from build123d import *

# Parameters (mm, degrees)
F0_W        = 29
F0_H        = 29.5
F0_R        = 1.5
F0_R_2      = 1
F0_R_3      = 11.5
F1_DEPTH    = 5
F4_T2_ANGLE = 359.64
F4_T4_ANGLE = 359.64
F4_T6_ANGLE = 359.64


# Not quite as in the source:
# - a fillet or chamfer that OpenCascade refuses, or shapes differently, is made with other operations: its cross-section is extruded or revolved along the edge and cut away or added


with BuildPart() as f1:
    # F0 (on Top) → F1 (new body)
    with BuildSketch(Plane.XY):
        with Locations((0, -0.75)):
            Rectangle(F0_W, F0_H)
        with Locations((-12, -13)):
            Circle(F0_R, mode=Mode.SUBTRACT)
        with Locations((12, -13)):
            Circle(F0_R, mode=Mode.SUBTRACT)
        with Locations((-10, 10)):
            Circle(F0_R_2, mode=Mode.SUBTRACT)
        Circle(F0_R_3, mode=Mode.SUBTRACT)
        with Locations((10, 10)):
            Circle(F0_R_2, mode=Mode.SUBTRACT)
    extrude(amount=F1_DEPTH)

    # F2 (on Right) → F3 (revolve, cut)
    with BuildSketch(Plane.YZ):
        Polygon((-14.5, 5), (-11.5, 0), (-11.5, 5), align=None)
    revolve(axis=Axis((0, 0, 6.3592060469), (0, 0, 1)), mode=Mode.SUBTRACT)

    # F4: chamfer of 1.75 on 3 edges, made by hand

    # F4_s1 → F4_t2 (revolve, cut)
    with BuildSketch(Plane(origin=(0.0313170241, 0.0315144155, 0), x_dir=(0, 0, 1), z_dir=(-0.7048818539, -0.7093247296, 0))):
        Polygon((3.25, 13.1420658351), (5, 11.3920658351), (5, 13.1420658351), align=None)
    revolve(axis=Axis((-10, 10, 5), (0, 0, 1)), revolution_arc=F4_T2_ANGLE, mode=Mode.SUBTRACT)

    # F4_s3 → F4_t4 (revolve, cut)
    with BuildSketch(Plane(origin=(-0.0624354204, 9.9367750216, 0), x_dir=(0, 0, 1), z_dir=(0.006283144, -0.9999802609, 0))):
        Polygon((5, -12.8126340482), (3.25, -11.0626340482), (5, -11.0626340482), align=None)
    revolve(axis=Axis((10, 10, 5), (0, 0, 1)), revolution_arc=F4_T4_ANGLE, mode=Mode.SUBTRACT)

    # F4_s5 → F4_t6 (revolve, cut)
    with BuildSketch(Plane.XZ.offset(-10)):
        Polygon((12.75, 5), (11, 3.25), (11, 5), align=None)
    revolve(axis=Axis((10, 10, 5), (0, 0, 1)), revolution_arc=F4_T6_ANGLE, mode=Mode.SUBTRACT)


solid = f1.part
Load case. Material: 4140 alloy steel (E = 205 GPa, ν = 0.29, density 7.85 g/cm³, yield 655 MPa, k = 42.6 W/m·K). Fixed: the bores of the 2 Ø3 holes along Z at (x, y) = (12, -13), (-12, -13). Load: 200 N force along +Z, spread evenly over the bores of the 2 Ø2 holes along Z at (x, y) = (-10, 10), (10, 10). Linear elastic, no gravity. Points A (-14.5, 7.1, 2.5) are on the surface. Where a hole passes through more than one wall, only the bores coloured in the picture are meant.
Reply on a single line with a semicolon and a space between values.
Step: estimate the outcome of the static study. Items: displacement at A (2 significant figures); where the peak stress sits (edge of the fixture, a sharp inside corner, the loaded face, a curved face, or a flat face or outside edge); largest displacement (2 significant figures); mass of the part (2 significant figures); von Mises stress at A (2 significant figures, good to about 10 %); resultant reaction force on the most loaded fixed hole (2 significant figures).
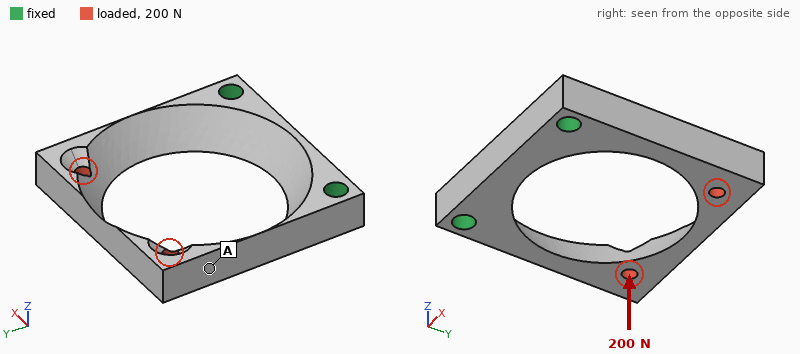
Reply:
0.057 mm; a sharp inside corner; 0.11 mm; 12 g; 29 MPa; 100 N
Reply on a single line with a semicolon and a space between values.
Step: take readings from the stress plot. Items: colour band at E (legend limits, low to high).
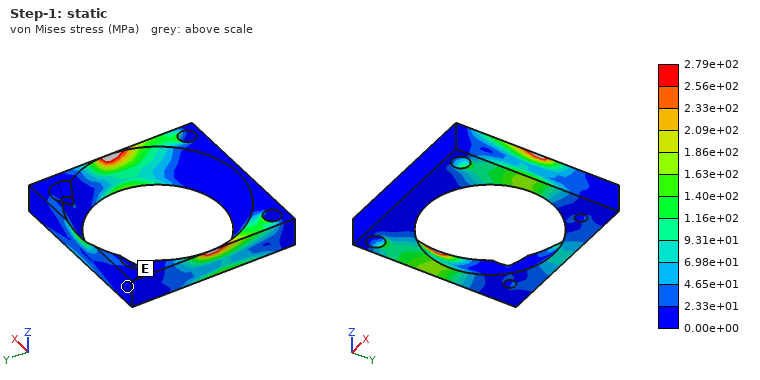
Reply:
0.00e+00 to 2.33e+01 MPa
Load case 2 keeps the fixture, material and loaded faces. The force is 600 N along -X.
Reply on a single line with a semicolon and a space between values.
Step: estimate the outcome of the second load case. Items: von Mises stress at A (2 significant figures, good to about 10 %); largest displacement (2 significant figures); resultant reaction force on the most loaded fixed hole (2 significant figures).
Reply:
140 MPa; 0.13 mm; 430 N
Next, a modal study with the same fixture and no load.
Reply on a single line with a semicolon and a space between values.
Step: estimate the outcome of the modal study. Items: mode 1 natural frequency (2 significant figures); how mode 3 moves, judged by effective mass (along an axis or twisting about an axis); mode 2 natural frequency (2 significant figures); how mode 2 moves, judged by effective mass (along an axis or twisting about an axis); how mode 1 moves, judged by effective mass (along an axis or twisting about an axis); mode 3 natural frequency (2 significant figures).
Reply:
3400 Hz; along X; 4700 Hz; along X; along Z; 6600 Hz
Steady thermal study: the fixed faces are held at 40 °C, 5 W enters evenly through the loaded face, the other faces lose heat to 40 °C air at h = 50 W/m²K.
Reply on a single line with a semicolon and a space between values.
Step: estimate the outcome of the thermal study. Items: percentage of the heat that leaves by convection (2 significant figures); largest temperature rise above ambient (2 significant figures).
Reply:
48 %; 68 K
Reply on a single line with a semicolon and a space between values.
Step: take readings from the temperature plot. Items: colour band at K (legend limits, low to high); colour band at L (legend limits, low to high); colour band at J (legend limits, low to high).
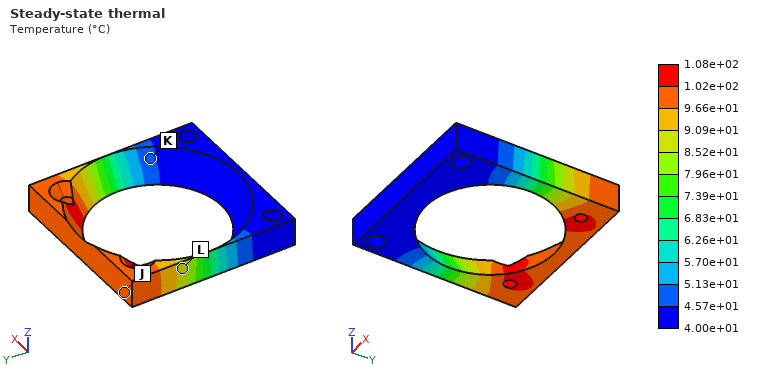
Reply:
4.57e+01 to 5.13e+01 °C; 8.52e+01 to 9.09e+01 °C; 9.66e+01 to 1.02e+02 °C
